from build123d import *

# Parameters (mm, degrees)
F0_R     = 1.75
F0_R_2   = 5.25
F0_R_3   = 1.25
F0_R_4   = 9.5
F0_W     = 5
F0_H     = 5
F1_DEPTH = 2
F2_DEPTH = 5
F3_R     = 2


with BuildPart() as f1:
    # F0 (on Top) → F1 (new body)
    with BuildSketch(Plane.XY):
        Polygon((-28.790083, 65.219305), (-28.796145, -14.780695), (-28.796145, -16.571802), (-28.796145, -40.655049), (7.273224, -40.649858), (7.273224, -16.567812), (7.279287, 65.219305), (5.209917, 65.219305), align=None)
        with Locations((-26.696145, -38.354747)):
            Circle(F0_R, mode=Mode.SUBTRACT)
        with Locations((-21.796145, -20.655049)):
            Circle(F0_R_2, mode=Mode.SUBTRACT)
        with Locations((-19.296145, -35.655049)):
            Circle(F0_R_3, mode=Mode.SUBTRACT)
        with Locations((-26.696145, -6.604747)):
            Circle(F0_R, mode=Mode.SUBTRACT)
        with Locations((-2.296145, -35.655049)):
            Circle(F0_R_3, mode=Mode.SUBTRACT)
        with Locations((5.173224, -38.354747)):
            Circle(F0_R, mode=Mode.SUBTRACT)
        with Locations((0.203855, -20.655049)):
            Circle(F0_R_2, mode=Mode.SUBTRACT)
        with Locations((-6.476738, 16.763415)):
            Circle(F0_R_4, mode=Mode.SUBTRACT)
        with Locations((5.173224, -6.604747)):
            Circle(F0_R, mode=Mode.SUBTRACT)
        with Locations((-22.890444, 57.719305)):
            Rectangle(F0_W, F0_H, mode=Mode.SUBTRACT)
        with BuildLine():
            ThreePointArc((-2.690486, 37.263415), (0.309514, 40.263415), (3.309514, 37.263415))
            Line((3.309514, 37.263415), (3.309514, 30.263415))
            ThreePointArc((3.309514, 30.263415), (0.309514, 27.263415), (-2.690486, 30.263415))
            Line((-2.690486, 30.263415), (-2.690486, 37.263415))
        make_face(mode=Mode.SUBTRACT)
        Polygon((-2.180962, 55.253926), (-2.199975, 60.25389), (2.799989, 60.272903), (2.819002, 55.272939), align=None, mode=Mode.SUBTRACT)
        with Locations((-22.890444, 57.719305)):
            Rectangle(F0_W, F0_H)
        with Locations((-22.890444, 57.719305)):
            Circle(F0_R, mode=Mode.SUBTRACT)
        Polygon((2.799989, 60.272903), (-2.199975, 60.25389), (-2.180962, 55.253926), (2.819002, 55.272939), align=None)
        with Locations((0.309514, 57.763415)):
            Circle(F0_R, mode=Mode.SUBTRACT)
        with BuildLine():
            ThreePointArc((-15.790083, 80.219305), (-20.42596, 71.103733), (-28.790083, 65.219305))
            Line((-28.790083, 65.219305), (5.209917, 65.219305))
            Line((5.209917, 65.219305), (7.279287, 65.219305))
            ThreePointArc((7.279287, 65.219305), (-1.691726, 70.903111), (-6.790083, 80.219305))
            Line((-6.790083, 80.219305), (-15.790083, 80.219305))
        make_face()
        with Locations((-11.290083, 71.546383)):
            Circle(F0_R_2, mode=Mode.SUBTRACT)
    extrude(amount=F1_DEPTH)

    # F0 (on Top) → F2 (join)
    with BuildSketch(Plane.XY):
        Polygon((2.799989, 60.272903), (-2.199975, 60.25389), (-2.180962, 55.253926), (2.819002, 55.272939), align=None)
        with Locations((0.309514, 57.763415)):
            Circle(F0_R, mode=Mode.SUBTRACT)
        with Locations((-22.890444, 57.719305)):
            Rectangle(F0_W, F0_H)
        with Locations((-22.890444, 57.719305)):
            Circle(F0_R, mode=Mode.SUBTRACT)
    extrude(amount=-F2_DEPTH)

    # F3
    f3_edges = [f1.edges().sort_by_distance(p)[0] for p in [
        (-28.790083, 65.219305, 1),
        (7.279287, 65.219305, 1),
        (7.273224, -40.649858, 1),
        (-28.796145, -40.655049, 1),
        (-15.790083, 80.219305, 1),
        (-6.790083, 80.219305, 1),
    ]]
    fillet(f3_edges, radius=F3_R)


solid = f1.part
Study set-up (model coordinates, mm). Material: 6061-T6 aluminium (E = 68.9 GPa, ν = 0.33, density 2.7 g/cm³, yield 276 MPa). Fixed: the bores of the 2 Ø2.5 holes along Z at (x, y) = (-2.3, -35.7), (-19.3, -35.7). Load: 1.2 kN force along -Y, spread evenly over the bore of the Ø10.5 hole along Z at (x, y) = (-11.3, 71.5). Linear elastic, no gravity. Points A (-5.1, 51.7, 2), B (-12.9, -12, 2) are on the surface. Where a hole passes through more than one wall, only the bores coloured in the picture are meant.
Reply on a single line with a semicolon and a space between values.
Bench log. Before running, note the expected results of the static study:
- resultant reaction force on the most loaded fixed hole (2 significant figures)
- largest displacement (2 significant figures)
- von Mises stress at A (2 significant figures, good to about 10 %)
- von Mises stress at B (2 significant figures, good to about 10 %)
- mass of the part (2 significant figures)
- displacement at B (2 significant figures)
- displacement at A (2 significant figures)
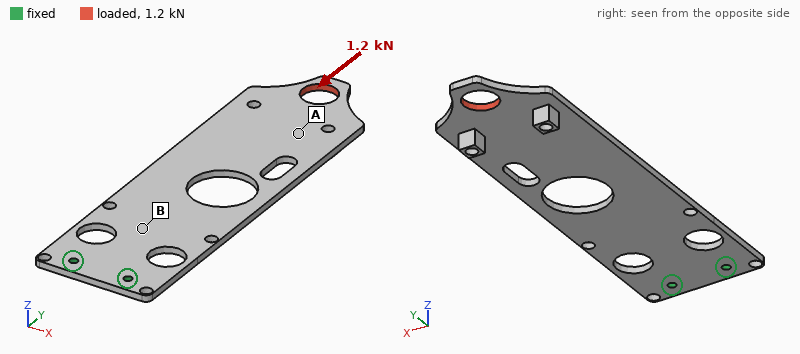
640 N; 60 µm; 16 MPa; 26 MPa; 19 g; 12 µm; 45 µm
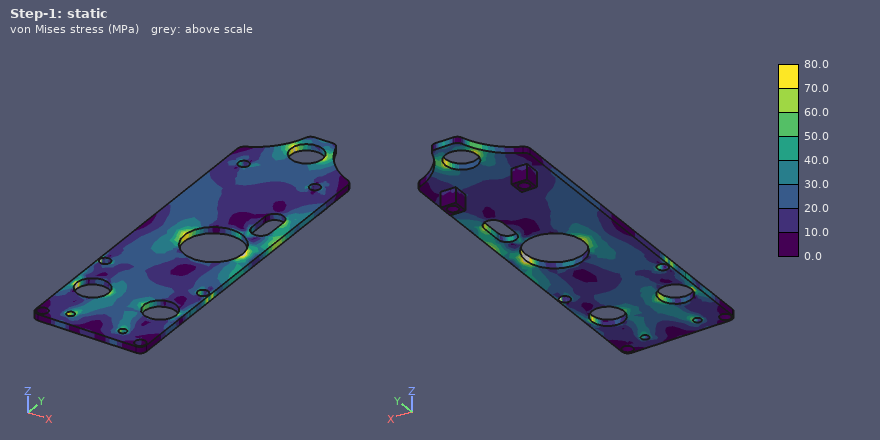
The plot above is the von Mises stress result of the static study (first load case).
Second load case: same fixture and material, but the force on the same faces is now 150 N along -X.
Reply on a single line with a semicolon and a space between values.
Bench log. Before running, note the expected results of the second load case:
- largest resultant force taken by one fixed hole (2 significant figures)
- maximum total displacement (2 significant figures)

860 N; 0.33 mm
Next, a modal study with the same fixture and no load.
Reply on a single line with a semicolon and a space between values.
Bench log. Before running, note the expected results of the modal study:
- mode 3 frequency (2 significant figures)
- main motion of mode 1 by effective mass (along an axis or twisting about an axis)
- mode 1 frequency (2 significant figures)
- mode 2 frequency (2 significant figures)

810 Hz; along Z; 120 Hz; 760 Hz
